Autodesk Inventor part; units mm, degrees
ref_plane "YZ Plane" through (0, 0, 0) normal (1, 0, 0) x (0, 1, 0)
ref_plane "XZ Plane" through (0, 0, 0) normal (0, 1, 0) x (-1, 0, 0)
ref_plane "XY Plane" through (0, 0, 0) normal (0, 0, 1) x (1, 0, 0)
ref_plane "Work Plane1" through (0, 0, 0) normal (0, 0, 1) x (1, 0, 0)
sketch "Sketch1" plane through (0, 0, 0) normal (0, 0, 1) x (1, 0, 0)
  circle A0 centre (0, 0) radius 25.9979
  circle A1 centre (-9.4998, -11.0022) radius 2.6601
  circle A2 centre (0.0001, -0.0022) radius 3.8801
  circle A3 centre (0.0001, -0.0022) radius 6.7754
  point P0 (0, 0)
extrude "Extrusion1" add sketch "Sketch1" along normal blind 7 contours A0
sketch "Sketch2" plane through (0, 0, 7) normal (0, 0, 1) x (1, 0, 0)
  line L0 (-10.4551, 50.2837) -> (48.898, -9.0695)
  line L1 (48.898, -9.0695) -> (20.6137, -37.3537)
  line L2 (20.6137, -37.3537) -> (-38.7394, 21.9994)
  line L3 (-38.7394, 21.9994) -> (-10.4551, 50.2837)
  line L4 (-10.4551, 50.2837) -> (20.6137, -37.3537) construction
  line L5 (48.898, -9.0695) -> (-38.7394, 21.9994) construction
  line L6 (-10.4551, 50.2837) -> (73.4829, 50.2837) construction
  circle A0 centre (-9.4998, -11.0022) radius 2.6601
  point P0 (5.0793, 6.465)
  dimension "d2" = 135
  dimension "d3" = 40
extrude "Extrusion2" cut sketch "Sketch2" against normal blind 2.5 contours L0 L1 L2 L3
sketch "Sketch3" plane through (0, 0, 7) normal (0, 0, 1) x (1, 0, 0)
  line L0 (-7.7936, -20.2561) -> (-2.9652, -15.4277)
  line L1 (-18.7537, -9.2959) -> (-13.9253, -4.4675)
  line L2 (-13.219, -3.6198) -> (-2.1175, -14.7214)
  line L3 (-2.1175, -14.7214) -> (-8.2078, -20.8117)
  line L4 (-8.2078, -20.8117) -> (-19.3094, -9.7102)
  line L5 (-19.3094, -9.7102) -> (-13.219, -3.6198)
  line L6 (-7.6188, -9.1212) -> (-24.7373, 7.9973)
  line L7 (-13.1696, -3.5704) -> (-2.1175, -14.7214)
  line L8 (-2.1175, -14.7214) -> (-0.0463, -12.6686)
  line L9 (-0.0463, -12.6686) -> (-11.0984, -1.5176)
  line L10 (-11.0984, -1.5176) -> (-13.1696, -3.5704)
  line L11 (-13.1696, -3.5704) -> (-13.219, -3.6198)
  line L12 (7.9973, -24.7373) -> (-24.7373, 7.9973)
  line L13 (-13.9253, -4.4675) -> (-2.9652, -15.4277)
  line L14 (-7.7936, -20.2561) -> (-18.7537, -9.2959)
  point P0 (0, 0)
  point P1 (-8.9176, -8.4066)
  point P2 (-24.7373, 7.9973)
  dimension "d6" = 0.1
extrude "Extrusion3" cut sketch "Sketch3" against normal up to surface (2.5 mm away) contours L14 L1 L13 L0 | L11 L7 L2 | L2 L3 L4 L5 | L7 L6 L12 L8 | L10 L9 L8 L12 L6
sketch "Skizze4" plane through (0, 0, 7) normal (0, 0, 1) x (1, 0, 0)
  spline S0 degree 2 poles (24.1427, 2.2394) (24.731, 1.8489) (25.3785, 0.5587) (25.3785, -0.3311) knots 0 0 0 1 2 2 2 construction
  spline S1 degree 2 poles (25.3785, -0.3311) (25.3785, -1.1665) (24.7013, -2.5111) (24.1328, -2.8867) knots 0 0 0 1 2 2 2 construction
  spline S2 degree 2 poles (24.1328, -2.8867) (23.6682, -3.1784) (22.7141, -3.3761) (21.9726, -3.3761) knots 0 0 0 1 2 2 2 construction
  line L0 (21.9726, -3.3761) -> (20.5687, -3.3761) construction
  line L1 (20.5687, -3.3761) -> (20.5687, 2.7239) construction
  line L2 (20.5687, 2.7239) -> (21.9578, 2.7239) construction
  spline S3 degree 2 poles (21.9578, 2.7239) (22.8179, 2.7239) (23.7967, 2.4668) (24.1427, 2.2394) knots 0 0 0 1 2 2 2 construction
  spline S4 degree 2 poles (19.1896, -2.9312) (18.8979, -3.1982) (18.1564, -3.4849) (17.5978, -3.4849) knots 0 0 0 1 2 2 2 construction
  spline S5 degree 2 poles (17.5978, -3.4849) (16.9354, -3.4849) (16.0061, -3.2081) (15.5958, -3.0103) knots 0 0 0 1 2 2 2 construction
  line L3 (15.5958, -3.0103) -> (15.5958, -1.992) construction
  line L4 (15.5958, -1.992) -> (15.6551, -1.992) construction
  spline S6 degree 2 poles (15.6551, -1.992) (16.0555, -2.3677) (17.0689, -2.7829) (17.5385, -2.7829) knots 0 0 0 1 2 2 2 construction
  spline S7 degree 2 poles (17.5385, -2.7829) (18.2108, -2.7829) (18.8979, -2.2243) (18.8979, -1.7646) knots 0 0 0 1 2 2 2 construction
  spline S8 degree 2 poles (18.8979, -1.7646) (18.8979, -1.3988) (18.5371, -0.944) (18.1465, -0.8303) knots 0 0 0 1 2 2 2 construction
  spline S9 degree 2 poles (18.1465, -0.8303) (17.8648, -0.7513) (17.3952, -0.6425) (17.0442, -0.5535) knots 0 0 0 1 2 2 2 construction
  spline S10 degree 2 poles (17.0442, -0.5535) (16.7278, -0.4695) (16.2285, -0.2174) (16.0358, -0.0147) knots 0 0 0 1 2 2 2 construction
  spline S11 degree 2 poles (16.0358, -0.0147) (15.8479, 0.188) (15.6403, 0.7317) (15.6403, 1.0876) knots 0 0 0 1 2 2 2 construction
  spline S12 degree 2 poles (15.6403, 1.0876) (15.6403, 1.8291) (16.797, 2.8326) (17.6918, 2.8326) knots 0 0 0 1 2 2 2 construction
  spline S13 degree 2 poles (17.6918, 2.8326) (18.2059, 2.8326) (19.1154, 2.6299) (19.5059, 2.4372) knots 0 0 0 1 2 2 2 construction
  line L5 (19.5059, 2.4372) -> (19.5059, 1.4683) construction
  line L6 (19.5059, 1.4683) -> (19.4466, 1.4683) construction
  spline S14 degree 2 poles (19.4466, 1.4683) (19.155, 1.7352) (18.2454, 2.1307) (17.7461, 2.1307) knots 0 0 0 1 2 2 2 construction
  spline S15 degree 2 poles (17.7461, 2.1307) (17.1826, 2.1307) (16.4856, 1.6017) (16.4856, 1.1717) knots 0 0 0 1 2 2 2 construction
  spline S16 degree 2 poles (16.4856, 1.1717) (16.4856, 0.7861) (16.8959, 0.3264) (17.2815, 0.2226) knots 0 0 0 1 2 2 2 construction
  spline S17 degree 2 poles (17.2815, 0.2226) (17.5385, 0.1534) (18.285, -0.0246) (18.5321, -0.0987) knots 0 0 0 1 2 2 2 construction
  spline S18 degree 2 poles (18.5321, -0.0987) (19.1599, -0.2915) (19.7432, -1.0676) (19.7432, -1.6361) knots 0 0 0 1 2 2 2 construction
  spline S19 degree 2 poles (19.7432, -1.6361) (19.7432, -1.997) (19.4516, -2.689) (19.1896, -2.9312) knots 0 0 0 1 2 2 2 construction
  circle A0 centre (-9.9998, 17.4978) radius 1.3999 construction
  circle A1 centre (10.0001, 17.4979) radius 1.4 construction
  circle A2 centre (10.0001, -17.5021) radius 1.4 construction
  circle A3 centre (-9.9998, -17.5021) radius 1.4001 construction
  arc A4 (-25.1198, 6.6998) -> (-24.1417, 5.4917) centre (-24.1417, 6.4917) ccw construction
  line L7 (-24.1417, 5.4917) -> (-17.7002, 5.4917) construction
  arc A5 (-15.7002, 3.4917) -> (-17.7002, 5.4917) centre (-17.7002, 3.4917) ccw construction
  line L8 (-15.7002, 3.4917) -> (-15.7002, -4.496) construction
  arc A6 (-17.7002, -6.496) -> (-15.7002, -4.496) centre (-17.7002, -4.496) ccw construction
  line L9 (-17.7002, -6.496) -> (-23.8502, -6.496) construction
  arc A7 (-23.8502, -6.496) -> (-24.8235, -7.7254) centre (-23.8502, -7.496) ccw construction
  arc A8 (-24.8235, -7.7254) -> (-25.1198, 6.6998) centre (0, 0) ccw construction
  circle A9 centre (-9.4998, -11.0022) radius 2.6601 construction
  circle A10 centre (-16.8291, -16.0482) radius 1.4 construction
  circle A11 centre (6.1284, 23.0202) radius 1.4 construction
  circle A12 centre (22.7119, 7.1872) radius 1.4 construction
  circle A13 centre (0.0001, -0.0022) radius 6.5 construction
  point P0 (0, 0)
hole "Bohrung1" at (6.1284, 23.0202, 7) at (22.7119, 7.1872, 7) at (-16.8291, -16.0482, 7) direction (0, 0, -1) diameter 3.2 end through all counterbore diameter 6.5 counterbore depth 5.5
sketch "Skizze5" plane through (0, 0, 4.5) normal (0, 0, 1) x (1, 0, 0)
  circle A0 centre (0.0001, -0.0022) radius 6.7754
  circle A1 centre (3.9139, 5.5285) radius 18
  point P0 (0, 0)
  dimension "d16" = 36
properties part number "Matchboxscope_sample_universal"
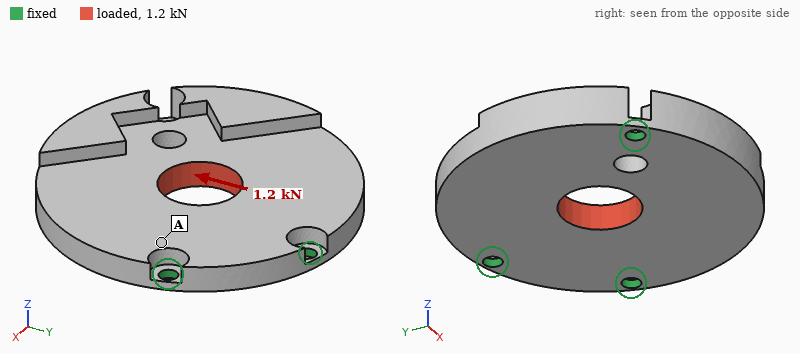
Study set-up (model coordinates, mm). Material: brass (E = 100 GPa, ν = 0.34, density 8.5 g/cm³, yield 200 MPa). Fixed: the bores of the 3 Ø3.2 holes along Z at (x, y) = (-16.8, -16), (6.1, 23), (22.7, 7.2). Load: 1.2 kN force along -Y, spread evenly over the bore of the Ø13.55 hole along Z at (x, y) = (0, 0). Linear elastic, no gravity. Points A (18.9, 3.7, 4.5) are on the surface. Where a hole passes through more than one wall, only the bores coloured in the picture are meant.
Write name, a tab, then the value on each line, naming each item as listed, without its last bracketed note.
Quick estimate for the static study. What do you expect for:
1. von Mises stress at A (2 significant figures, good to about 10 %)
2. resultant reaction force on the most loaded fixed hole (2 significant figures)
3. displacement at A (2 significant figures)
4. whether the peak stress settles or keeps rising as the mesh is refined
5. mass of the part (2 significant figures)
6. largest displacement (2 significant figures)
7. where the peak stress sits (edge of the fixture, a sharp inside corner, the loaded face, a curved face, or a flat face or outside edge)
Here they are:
von Mises stress at A	8.2 MPa
resultant reaction force on the most loaded fixed hole	460 N
displacement at A	2.5 µm
whether the peak stress settles or keeps rising as the mesh is refined	keeps rising
mass of the part	79 g
largest displacement	9.4 µm
where the peak stress sits	edge of the fixture
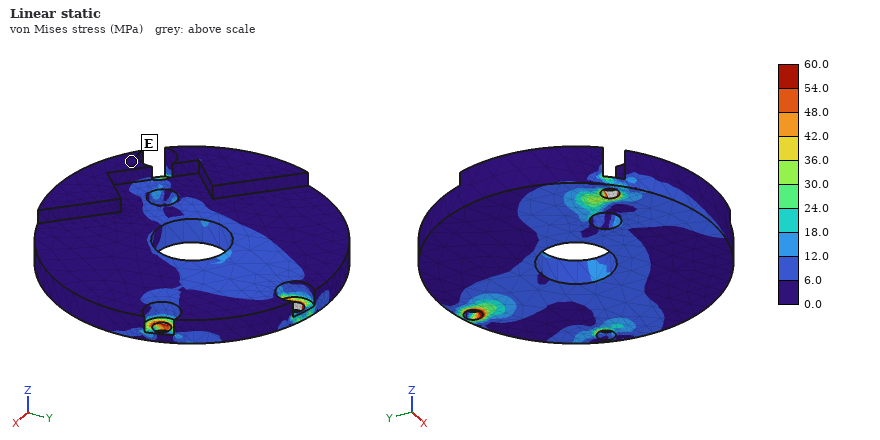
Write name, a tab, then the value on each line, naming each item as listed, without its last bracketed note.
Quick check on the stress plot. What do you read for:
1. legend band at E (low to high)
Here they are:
legend band at E	0.0 to 6.0 MPa
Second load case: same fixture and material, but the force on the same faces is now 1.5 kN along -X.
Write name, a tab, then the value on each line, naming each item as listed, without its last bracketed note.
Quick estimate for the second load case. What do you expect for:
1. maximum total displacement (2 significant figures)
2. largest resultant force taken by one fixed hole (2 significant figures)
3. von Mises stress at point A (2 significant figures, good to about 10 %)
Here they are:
maximum total displacement	11 µm
largest resultant force taken by one fixed hole	580 N
von Mises stress at point A	14 MPa
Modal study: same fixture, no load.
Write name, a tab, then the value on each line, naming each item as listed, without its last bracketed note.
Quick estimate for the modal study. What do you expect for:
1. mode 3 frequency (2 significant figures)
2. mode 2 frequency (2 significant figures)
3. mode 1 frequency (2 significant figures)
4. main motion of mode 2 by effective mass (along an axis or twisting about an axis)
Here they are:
mode 3 frequency	8000 Hz
mode 2 frequency	3500 Hz
mode 1 frequency	2600 Hz
main motion of mode 2 by effective mass	along Z
